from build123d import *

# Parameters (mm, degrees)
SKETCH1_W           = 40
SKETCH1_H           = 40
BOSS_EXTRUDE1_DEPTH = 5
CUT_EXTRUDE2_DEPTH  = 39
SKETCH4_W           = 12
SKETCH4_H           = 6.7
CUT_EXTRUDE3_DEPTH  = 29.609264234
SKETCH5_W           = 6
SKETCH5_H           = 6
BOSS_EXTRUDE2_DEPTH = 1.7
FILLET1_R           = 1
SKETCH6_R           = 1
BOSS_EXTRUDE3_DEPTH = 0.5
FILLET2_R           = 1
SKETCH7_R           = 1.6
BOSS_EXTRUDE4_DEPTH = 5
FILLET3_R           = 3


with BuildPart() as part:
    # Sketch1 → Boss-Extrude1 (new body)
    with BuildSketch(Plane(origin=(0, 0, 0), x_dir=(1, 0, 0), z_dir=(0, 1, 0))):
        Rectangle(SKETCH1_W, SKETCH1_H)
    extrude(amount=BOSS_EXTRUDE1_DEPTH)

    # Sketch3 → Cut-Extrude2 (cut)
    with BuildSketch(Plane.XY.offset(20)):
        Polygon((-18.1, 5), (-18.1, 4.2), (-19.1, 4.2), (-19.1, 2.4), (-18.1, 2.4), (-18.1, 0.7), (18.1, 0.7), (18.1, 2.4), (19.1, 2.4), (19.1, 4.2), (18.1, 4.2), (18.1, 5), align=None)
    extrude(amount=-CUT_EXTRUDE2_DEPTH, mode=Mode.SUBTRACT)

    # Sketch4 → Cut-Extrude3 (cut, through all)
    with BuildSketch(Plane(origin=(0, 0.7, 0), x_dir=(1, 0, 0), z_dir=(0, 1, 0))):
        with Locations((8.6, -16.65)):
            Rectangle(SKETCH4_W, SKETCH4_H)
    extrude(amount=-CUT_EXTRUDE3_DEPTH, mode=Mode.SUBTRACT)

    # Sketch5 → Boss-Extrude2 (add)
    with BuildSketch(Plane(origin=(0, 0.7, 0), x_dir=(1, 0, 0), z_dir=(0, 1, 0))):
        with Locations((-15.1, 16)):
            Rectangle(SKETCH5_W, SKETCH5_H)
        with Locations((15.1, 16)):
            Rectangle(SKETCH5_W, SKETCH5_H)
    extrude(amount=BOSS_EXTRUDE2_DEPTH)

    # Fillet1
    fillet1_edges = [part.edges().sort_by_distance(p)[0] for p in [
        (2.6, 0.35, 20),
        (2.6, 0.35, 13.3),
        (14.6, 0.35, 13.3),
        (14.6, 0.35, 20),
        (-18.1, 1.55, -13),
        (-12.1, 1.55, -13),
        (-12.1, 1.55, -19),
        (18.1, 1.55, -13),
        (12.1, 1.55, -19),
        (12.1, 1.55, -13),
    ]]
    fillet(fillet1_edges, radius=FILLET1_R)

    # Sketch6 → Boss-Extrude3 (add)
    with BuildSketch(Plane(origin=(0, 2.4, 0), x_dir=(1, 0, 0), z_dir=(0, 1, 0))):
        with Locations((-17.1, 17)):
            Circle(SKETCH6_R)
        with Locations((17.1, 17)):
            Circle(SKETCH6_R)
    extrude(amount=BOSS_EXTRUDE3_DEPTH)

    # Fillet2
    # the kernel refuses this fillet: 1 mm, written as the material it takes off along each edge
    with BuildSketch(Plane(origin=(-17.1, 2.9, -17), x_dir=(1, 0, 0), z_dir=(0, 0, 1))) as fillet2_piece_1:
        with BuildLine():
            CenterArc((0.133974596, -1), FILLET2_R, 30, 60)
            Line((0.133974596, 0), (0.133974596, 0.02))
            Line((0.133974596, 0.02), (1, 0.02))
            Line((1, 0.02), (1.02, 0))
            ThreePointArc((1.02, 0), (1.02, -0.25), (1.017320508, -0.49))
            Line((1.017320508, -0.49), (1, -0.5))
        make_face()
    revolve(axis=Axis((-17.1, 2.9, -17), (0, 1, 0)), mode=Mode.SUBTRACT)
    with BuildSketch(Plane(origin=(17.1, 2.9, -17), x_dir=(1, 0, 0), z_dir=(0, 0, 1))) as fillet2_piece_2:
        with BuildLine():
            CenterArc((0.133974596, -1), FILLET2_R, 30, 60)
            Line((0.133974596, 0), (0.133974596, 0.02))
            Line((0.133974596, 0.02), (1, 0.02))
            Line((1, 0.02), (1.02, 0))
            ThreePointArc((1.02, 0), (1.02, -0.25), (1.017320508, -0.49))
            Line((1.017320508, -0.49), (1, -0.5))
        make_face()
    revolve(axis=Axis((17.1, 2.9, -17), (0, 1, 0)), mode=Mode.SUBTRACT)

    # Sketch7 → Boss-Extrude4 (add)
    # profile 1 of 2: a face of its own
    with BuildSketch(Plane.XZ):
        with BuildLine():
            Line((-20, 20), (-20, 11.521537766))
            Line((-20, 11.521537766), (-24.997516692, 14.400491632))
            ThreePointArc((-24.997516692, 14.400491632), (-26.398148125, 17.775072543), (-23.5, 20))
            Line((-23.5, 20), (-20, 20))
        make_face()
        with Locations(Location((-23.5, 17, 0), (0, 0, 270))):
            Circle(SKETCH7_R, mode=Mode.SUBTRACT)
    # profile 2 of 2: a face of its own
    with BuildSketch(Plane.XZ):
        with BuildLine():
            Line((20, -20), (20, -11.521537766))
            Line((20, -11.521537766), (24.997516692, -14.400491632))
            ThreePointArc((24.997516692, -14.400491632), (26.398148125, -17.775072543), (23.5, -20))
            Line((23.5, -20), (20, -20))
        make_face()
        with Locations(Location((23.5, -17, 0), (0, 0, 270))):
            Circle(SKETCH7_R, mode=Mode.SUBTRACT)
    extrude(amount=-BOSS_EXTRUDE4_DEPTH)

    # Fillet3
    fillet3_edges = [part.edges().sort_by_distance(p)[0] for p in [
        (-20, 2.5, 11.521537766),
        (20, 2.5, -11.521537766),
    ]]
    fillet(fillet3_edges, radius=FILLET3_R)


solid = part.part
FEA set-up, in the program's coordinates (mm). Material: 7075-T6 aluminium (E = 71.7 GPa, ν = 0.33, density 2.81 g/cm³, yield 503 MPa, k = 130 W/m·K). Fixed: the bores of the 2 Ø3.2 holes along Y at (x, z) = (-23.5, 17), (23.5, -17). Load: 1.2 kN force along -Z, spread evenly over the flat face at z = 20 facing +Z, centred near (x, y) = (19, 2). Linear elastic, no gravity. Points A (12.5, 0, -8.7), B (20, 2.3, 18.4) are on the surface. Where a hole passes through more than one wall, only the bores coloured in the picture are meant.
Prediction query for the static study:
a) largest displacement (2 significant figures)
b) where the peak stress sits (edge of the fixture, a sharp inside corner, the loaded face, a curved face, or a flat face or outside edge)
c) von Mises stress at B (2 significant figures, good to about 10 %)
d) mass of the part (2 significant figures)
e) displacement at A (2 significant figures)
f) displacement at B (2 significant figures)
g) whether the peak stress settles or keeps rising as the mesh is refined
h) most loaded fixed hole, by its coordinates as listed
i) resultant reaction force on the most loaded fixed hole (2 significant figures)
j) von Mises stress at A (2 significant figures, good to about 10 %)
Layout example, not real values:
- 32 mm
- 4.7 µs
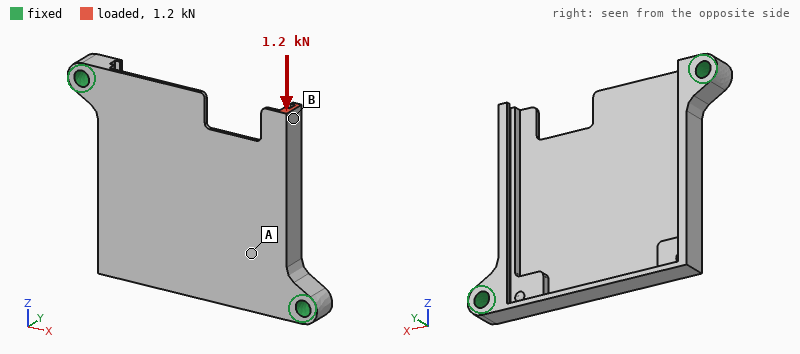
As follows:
- 92 µm
- edge of the fixture
- 130 MPa
- 6.1 g
- 22 µm
- 83 µm
- keeps rising
- (23.5, -17)
- 1.1 kN
- 16 MPa
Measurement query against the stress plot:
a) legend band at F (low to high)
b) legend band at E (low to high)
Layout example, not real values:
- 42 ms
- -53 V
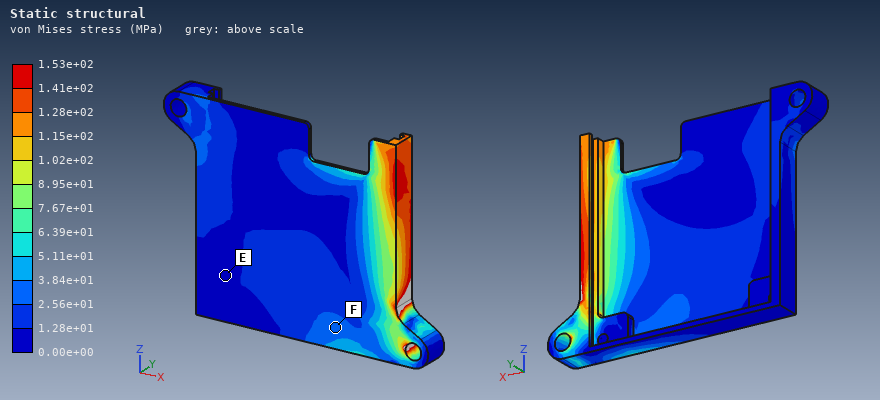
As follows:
- 2.56e+01 to 3.84e+01 MPa
- 0.00e+00 to 1.28e+01 MPa
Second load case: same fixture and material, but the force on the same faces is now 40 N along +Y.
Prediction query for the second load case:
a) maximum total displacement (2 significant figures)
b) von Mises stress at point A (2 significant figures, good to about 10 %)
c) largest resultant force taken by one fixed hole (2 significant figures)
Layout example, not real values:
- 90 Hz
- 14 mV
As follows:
- 0.31 mm
- 30 MPa
- 95 N
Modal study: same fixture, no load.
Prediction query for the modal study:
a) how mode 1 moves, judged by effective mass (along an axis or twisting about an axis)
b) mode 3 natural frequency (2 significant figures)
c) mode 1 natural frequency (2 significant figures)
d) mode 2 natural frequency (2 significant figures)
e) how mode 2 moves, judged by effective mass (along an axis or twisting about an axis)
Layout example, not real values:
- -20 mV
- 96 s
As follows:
- along Y
- 3800 Hz
- 2300 Hz
- 3100 Hz
- along Y
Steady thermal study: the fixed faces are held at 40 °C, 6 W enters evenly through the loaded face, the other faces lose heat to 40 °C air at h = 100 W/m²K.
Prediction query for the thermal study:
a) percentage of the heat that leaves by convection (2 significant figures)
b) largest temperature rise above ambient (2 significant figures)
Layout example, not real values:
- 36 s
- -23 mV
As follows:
- 62 %
- 76 K
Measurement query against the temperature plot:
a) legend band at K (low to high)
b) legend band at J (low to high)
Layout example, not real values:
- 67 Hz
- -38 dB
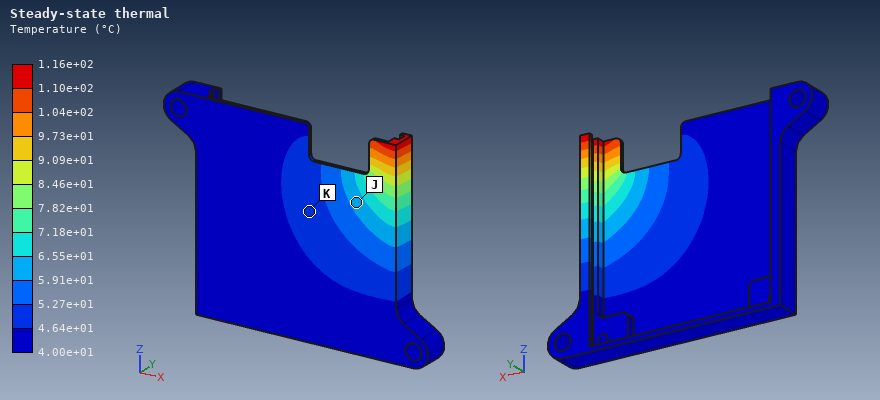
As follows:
- 4.64e+01 to 5.27e+01 °C
- 5.91e+01 to 6.55e+01 °C
